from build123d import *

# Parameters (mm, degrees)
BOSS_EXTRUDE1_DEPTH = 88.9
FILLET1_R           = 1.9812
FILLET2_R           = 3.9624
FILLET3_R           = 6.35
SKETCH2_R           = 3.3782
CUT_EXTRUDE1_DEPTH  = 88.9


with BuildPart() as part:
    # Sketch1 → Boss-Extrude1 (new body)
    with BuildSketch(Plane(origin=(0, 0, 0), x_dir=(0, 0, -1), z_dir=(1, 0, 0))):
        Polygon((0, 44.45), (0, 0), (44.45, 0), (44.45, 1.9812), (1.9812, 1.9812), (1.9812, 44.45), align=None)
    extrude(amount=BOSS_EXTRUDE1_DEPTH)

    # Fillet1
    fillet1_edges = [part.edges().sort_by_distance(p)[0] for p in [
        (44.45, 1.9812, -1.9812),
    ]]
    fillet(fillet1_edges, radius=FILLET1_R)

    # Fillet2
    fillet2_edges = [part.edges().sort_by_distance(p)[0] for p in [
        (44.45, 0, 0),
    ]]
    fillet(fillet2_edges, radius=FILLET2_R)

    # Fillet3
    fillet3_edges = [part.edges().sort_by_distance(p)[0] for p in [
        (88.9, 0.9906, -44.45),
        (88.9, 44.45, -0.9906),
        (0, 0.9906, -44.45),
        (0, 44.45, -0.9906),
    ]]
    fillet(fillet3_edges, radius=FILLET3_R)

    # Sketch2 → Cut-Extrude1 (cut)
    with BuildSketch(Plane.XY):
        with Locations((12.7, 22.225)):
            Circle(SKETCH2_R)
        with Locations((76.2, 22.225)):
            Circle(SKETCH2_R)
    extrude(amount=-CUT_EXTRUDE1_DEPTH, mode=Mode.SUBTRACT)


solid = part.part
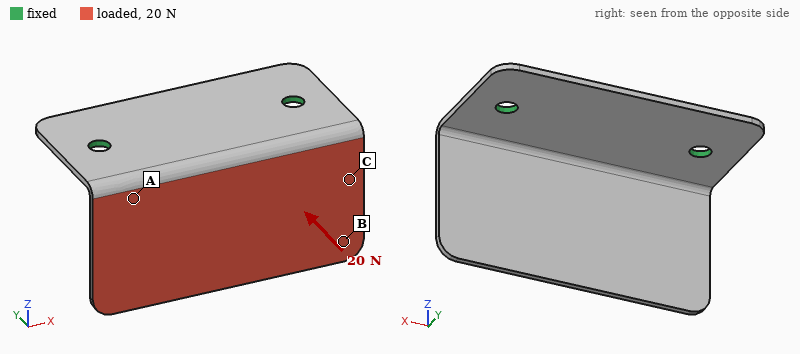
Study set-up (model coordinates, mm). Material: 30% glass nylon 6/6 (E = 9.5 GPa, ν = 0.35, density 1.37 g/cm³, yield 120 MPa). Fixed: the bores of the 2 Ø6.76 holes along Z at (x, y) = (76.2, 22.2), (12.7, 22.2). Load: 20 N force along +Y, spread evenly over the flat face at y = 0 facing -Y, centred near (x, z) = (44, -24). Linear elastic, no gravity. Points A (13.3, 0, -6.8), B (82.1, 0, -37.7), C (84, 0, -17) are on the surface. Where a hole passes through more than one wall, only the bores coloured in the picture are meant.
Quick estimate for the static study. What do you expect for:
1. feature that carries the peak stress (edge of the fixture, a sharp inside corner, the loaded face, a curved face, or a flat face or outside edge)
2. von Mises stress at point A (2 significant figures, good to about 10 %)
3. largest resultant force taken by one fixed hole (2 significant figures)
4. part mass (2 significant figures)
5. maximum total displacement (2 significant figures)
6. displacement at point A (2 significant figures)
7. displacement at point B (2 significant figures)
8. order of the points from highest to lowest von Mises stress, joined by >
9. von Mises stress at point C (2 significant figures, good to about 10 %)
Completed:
a flat face or outside edge
5.1 MPa
10 N
20 g
1.1 mm
0.23 mm
0.88 mm
A > C > B
2.9 MPa
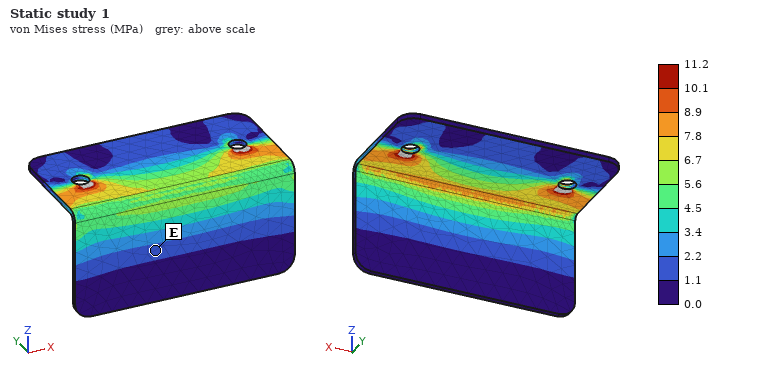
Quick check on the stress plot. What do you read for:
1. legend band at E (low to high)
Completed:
1.1 to 2.2 MPa
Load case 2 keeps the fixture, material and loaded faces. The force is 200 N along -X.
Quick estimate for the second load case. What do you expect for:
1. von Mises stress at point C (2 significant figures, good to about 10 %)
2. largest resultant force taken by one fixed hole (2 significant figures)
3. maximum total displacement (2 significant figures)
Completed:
8.2 MPa
140 N
1.3 mm
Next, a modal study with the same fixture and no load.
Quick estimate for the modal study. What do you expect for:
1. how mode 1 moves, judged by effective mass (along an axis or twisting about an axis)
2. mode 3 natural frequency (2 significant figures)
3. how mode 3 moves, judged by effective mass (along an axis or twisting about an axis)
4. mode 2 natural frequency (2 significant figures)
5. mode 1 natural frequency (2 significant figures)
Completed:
along Y
860 Hz
along Z
490 Hz
260 Hz
